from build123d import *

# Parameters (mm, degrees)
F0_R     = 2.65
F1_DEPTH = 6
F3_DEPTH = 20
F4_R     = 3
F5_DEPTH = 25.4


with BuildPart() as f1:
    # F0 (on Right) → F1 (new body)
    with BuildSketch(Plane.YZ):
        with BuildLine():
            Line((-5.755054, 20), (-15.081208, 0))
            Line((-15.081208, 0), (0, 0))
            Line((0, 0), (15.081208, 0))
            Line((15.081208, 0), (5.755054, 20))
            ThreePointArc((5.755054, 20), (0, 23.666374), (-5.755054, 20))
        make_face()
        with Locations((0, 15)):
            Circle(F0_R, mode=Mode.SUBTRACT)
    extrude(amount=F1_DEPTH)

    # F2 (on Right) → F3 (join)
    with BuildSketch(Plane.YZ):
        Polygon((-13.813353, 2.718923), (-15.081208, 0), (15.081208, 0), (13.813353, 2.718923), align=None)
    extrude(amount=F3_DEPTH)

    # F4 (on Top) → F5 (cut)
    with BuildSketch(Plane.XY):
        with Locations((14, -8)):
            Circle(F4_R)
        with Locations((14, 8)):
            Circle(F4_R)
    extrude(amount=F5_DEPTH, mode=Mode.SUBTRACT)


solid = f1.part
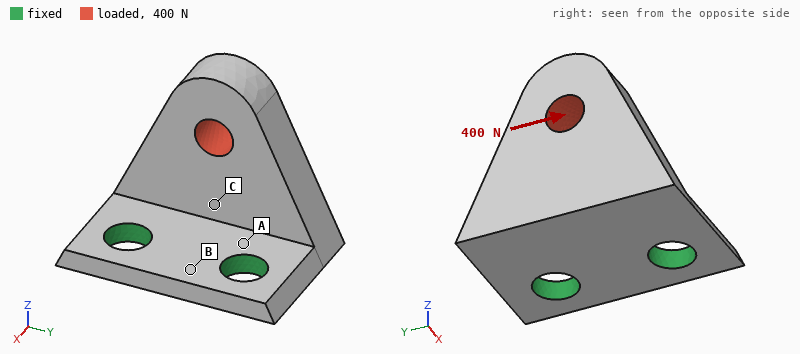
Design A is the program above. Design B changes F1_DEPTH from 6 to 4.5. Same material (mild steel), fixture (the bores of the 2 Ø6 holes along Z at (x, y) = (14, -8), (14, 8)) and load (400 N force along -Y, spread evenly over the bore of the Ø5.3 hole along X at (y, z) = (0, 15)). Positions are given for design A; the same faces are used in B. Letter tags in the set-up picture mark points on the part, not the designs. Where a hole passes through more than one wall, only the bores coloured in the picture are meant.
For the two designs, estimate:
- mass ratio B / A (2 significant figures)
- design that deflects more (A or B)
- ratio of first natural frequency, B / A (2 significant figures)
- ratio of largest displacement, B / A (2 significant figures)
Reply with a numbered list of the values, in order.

1. 0.85
2. B
3. 1.0
4. 1.6
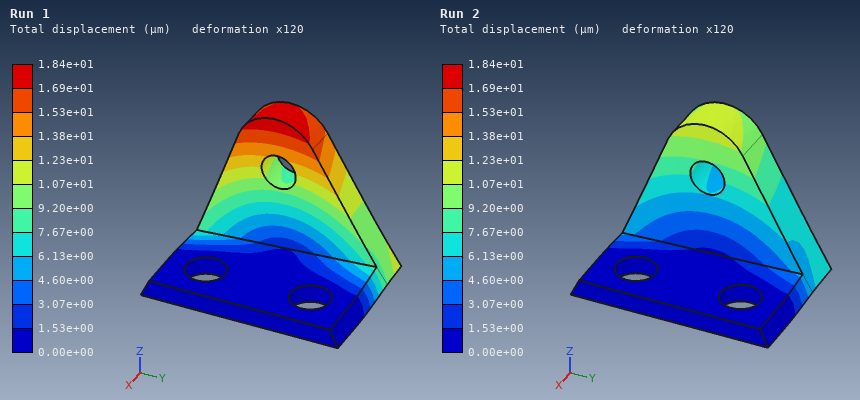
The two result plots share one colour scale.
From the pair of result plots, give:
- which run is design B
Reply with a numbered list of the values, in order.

1. Run 1
